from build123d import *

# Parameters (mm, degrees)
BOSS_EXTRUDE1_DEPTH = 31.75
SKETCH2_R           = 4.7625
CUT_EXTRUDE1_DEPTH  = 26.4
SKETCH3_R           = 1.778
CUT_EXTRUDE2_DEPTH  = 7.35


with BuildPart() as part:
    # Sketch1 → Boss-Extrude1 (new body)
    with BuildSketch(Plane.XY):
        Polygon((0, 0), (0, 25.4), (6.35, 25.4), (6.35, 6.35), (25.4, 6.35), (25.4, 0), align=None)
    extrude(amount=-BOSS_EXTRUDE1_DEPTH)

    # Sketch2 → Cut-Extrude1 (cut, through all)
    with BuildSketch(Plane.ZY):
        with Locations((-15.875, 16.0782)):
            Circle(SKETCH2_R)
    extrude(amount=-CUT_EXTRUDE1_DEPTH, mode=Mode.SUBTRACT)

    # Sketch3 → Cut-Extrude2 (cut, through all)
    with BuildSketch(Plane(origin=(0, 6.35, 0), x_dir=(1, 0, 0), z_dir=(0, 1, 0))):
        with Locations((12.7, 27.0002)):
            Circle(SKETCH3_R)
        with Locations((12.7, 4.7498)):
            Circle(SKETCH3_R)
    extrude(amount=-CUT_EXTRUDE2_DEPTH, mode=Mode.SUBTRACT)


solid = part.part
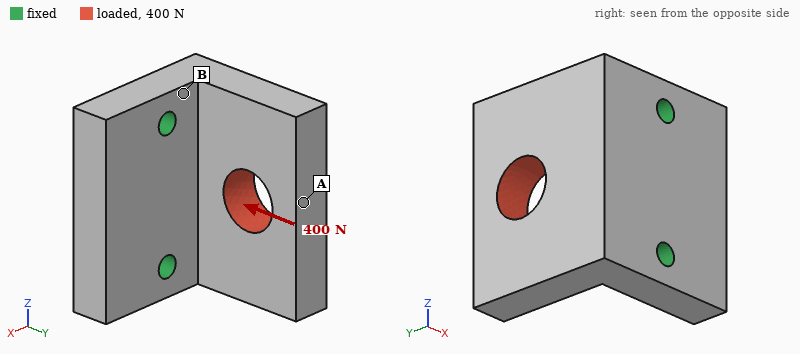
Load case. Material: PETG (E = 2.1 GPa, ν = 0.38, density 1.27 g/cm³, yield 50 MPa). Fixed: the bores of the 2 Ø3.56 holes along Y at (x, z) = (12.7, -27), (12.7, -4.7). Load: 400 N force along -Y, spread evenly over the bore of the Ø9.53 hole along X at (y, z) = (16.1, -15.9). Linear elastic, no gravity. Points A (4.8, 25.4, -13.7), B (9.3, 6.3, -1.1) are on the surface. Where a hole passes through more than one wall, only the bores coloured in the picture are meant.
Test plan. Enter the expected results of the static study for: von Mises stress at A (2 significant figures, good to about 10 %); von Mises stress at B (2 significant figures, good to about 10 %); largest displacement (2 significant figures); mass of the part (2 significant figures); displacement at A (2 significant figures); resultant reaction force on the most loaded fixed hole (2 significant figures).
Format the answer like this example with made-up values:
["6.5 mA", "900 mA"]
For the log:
["4.3 MPa", "11 MPa", "0.40 mm", "11 g", "0.37 mm", "200 N"]
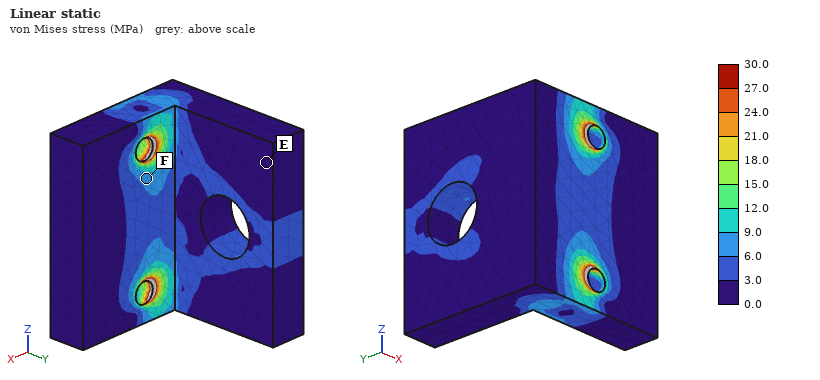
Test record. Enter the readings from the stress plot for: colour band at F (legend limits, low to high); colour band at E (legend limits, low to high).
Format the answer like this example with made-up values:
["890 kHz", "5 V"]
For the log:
["6.0 to 9.0 MPa", "0.0 to 3.0 MPa"]
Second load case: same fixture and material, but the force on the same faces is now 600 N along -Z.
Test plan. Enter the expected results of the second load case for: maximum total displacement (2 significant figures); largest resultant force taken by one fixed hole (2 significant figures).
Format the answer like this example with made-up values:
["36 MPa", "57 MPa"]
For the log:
["0.44 mm", "490 N"]
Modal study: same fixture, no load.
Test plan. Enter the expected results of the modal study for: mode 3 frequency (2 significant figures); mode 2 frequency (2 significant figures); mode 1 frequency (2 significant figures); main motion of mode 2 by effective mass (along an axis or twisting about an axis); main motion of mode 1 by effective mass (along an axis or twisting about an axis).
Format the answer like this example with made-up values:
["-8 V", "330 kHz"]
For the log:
["4100 Hz", "3000 Hz", "1600 Hz", "along Z", "along X"]
